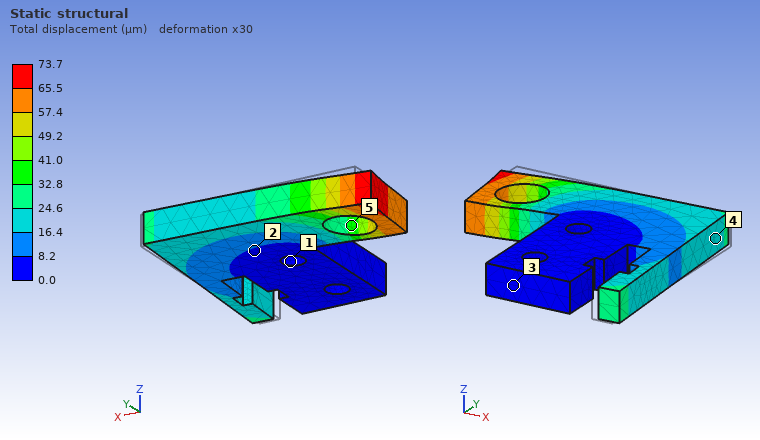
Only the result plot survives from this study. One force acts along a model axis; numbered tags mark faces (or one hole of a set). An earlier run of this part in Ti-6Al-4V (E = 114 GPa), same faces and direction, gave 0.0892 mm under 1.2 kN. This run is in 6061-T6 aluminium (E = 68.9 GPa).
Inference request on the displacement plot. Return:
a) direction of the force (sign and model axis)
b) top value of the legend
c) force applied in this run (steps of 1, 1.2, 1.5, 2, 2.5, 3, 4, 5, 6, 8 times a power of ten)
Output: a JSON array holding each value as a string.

["-Y", "73.7 µm", "600 N"]
